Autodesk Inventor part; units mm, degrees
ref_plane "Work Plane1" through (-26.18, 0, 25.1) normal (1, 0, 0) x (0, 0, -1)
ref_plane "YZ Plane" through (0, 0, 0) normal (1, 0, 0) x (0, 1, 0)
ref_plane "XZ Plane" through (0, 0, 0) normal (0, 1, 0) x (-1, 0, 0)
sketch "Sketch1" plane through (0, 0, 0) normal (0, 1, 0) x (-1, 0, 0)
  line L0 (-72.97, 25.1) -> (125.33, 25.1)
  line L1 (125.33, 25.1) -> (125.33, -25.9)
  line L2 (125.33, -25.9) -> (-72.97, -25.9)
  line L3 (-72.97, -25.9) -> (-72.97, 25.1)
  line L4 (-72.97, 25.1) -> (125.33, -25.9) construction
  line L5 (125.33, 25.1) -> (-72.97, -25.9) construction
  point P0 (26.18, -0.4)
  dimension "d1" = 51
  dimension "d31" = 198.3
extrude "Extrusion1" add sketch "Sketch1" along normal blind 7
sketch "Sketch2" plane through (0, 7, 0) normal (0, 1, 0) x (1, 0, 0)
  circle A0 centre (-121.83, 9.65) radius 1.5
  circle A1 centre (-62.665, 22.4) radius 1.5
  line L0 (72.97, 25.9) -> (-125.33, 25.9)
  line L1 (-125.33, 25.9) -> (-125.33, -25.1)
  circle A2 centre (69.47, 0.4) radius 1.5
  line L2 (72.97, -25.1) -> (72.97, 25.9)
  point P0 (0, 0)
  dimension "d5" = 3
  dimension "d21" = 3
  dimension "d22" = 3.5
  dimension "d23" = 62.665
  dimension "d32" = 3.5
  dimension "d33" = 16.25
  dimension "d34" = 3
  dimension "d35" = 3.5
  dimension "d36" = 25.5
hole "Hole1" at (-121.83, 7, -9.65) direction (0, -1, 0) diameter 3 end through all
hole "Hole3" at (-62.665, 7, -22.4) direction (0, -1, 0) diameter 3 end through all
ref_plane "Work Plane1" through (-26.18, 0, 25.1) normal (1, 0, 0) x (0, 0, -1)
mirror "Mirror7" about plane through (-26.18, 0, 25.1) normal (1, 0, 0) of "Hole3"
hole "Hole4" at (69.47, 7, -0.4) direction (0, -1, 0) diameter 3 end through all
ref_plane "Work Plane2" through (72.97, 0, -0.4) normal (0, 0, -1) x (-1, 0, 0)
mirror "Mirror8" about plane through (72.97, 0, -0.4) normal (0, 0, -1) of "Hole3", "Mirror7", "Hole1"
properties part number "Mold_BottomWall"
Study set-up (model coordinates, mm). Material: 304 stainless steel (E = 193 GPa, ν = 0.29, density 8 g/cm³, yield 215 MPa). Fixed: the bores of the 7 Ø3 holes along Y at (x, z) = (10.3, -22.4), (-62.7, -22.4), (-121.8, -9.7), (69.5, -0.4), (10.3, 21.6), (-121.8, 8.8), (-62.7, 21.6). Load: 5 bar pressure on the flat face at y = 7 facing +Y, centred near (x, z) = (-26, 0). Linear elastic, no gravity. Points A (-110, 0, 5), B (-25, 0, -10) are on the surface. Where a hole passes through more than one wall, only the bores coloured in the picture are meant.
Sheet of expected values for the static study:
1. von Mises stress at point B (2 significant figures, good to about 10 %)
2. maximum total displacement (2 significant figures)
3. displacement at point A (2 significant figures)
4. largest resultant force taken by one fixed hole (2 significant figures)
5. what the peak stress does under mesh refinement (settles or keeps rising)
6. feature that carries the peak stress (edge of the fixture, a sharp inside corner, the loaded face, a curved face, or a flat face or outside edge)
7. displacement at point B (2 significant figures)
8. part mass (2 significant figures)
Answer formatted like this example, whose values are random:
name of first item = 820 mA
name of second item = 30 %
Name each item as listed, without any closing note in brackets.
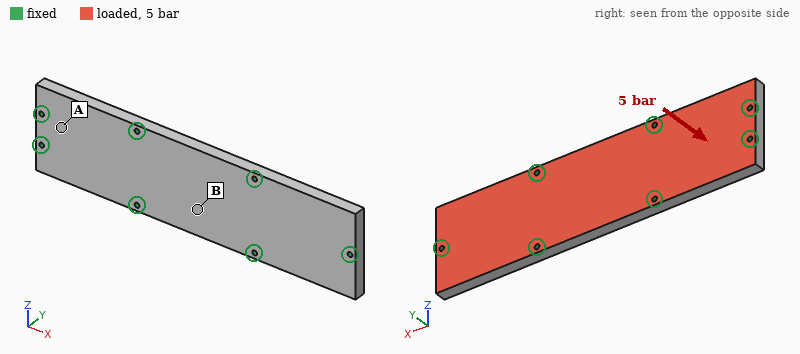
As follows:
von Mises stress at point B = 13 MPa
maximum total displacement = 9.7 µm
displacement at point A = 2.4 µm
largest resultant force taken by one fixed hole = 880 N
what the peak stress does under mesh refinement = keeps rising
feature that carries the peak stress = edge of the fixture
displacement at point B = 9.5 µm
part mass = 560 g
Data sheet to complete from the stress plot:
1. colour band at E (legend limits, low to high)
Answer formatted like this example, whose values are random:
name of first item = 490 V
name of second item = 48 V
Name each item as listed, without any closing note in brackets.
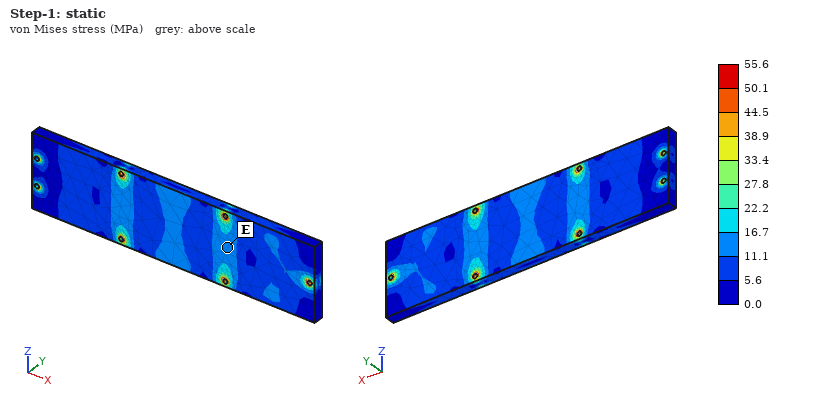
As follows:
colour band at E = 11.1 to 16.7 MPa
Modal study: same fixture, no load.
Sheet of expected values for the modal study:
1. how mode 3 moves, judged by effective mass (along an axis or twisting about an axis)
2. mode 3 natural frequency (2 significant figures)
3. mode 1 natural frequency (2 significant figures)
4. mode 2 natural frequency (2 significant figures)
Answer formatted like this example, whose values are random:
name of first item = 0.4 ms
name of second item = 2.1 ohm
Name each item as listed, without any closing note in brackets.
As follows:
how mode 3 moves, judged by effective mass = along Y
mode 3 natural frequency = 6400 Hz
mode 1 natural frequency = 5100 Hz
mode 2 natural frequency = 6100 Hz
